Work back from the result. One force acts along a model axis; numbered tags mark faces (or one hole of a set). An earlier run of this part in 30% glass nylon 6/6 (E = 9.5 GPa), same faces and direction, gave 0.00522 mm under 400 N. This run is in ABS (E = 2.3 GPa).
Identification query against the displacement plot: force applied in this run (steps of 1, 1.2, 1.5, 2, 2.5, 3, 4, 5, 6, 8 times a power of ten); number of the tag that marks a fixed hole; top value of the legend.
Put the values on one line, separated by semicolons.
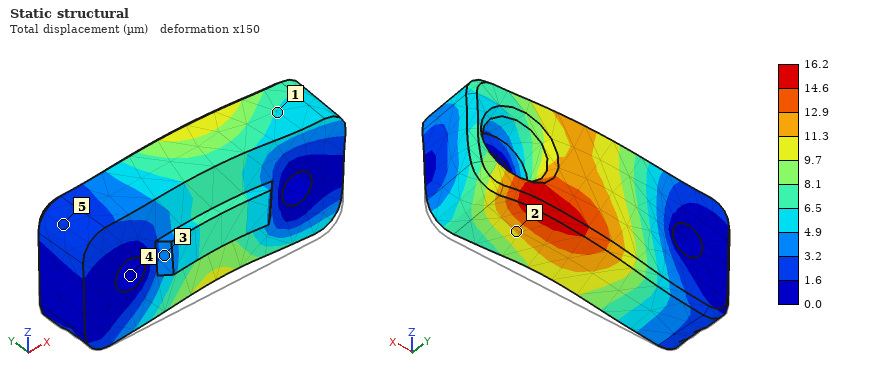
300 N; 4; 16.2 µm
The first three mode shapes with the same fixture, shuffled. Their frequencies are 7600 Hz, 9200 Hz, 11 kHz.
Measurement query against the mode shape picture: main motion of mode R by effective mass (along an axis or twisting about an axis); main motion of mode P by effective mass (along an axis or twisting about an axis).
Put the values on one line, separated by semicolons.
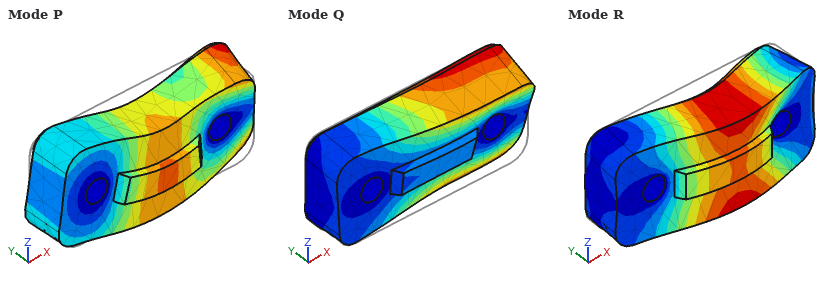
along Y; along Z
